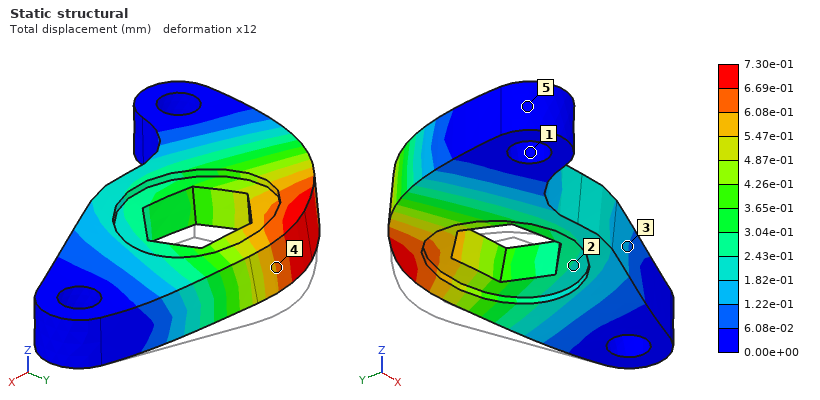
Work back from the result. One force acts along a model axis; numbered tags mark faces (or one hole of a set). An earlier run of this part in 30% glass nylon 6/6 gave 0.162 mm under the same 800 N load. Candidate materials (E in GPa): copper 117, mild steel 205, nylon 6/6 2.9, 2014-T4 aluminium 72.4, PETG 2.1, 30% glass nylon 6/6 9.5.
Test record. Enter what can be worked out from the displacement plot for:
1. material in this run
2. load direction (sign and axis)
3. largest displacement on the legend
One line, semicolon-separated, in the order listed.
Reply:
PETG; +Z; 7.30e-01 mm
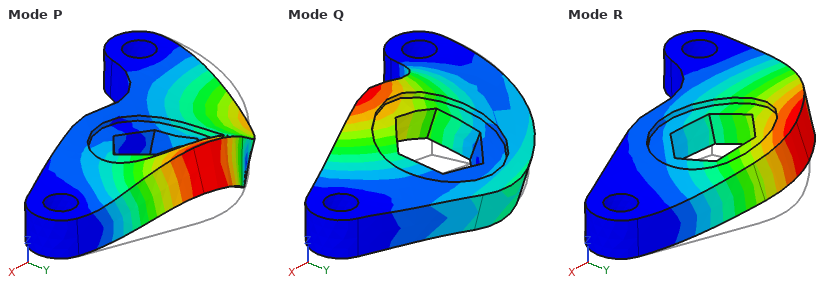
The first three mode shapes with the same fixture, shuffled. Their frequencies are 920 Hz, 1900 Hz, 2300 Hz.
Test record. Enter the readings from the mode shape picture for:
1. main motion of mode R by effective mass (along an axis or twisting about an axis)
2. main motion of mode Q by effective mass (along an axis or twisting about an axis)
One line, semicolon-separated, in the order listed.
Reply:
along Z; along Z
